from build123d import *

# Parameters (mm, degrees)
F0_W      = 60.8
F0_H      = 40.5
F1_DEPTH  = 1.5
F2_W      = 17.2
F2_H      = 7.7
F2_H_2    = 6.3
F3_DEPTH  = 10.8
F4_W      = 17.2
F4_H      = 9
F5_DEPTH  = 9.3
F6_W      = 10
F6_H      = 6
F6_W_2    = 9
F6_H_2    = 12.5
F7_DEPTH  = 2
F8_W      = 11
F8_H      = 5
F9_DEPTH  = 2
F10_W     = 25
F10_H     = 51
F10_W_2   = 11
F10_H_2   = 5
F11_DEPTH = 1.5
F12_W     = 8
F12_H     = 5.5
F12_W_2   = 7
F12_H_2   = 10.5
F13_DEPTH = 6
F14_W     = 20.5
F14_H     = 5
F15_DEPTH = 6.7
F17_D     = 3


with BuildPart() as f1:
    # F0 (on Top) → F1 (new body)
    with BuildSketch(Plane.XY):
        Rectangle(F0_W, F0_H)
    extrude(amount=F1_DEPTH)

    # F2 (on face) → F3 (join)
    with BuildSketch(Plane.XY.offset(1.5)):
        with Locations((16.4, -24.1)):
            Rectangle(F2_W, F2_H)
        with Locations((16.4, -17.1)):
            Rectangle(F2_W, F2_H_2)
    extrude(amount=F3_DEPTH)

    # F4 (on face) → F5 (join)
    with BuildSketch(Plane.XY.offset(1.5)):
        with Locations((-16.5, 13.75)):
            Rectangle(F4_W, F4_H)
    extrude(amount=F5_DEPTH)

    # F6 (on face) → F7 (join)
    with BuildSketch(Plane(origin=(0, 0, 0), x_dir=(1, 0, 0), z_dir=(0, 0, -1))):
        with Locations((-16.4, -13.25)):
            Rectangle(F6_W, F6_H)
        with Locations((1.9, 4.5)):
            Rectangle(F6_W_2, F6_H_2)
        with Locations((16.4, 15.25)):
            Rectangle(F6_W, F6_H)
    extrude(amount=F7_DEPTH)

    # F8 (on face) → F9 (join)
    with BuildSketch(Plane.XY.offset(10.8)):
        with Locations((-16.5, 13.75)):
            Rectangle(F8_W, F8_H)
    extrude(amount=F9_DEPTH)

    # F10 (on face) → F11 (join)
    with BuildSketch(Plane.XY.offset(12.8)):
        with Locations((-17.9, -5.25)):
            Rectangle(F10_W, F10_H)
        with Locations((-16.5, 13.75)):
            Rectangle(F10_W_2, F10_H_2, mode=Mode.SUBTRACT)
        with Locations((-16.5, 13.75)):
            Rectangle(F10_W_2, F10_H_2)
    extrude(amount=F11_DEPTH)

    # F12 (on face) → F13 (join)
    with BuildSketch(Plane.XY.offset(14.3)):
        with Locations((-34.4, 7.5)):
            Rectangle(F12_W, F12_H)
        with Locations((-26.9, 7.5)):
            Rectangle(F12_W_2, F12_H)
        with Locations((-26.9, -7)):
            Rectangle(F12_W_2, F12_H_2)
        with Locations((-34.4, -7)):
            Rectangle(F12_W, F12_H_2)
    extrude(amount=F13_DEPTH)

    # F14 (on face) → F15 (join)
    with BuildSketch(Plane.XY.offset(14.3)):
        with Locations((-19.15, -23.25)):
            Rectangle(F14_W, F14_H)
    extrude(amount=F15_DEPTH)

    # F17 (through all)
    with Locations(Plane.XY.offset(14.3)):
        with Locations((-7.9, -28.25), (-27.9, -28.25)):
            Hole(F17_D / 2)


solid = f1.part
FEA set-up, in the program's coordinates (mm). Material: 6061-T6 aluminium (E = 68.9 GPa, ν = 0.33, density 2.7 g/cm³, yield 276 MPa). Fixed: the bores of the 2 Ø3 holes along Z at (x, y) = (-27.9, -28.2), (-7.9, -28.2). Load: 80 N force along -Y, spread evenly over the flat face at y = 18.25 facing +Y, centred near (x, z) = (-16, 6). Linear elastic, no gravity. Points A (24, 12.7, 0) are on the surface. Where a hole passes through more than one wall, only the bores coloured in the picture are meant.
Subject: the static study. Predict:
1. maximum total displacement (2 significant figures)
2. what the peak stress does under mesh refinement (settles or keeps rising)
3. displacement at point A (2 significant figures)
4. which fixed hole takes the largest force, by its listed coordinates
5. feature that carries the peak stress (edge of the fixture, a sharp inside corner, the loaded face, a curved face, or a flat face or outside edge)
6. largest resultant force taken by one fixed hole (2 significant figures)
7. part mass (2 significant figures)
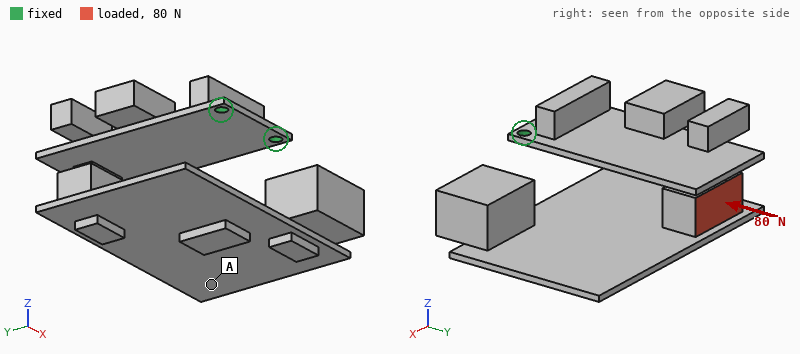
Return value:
1.1 mm
keeps rising
0.83 mm
(-7.9, -28.2)
edge of the fixture
50 N
33 g
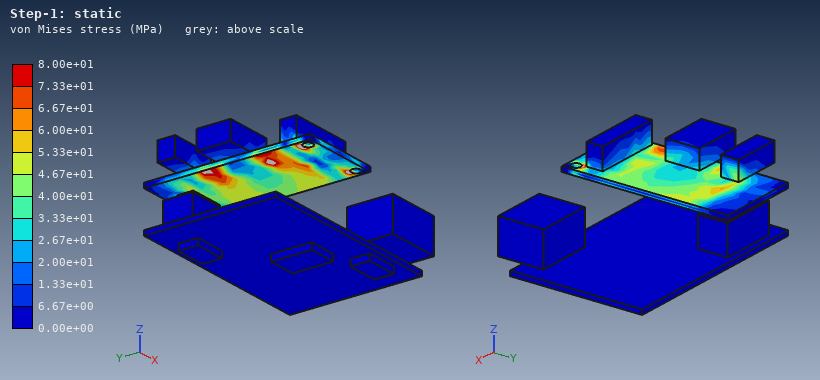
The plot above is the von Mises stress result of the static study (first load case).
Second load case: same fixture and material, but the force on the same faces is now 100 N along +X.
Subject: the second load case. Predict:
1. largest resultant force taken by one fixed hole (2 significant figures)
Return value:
240 N
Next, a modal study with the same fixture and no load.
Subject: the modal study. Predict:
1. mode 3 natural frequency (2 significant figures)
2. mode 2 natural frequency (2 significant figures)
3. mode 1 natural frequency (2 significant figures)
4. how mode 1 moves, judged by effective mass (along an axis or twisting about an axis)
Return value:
520 Hz
210 Hz
180 Hz
along Z
